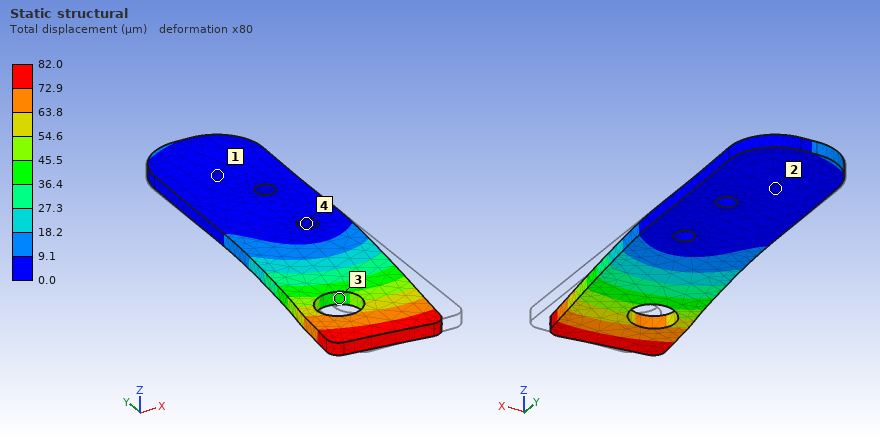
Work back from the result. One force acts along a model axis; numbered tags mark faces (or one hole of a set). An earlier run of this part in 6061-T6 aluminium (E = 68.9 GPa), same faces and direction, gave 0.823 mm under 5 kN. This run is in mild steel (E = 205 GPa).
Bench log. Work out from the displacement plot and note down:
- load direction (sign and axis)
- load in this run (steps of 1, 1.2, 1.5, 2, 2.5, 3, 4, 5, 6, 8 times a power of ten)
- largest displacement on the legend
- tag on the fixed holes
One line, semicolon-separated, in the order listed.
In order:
-X; 1.5 kN; 82.0 µm; 4
